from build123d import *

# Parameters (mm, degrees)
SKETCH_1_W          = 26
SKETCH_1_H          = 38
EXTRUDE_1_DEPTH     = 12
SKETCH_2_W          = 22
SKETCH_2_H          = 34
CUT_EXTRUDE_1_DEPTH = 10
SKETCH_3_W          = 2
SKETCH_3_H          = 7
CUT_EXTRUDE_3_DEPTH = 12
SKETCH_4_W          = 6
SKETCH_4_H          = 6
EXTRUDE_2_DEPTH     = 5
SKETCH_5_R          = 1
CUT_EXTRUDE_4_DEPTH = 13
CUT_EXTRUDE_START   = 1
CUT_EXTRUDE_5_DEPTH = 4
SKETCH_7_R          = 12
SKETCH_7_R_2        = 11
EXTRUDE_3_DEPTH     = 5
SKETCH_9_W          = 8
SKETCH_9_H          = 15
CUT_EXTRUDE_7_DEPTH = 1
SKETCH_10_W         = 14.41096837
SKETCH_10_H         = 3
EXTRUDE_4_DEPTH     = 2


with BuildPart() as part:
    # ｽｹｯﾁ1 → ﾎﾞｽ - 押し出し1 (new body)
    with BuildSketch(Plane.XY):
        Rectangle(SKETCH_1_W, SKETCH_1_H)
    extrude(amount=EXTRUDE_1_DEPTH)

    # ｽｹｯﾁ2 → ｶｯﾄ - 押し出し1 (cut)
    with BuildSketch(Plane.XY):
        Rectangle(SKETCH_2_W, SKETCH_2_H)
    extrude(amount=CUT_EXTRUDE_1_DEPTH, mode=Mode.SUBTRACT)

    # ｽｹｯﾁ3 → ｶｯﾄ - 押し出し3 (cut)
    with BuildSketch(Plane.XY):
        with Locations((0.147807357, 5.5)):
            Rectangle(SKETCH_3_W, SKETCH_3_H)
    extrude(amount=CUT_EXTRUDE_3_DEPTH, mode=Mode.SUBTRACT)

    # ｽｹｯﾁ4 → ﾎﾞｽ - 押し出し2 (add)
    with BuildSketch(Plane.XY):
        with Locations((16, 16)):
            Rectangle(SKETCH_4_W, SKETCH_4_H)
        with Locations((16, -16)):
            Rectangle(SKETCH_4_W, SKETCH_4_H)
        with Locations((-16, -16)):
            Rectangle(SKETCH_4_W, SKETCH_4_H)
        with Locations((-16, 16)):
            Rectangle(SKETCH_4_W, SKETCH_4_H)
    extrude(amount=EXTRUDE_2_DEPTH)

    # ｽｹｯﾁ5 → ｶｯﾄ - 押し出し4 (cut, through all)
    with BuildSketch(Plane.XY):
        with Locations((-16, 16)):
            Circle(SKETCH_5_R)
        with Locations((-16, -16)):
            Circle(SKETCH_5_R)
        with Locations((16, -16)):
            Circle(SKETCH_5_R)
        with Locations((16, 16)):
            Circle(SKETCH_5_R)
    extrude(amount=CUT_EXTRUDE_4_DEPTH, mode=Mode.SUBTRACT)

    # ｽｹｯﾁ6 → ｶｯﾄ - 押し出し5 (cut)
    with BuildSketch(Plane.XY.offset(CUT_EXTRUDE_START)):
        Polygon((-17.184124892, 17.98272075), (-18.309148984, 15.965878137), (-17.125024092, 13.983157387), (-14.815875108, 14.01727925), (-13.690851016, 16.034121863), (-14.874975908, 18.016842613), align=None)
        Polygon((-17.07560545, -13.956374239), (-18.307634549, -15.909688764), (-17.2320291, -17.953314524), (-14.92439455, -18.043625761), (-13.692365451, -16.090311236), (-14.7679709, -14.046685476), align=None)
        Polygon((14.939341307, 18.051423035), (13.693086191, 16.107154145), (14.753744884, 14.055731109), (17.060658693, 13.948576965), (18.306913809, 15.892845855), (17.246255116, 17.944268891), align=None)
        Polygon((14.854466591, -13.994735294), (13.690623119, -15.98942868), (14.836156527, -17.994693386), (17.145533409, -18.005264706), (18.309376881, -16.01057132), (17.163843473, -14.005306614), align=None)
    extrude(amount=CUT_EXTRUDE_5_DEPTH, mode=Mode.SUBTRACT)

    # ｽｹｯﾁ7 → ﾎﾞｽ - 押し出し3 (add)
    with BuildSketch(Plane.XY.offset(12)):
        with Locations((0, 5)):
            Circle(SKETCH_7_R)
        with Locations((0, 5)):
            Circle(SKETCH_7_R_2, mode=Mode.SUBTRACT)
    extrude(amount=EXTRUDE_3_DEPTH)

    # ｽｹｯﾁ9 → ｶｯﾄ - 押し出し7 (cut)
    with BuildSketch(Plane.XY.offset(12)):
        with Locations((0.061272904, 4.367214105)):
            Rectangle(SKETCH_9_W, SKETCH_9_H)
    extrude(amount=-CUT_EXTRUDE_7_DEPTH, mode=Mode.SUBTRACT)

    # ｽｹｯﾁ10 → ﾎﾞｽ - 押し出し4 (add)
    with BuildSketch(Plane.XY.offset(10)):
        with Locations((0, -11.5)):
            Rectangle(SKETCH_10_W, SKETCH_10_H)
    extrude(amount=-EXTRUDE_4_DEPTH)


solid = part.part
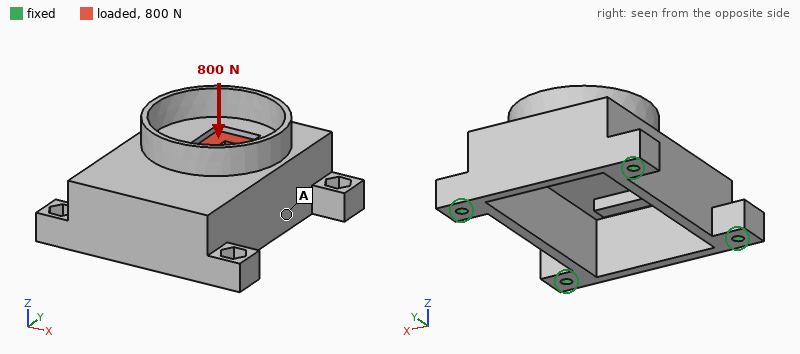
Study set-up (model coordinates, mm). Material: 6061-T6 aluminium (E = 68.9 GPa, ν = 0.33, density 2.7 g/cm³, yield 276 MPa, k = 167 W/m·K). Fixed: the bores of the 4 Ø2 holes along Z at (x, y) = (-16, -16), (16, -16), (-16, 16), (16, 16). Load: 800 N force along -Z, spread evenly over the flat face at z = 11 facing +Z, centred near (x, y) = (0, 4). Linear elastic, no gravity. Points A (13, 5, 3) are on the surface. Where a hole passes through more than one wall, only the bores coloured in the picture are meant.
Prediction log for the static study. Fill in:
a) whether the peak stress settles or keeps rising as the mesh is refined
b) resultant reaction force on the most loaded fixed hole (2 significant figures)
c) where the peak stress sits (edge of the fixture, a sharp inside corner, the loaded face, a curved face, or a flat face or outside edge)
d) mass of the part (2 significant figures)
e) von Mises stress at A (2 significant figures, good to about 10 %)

keeps rising
320 N
a sharp inside corner
14 g
22 MPa
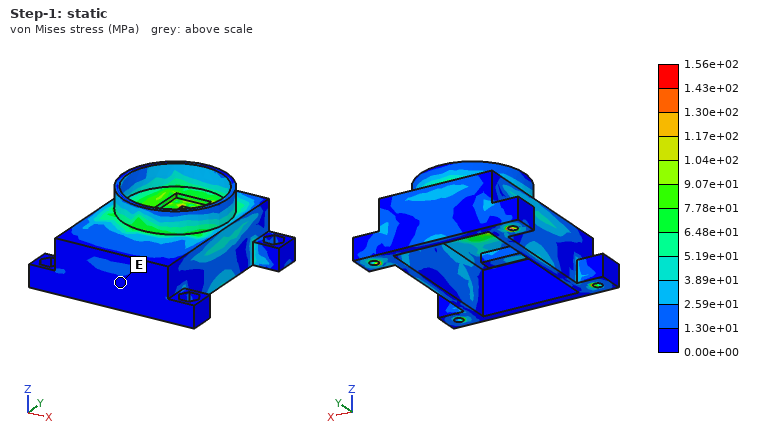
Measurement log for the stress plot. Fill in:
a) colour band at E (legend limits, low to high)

0.00e+00 to 1.30e+01 MPa
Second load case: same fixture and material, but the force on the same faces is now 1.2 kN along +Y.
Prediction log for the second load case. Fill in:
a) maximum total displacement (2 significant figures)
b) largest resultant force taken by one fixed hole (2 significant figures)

25 µm
360 N
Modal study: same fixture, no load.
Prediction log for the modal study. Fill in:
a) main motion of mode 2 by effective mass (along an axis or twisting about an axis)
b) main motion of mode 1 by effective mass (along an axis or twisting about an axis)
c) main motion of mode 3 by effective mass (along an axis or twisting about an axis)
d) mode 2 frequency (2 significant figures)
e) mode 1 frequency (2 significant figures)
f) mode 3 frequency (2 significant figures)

along Z
along Y
along X
13 kHz
12 kHz
15 kHz
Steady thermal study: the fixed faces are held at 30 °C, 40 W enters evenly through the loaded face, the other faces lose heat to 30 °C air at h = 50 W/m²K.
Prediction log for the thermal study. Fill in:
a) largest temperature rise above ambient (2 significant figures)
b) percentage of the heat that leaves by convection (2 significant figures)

59 K
19 %
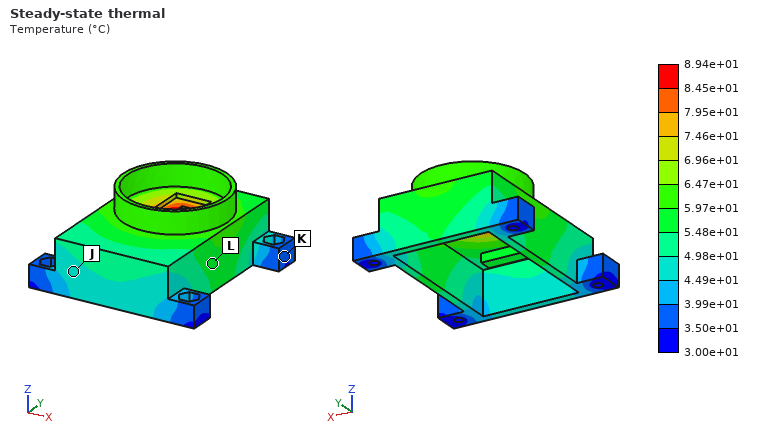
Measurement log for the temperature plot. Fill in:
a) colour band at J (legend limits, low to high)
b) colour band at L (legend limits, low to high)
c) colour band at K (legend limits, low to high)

4.49e+01 to 4.98e+01 °C
5.48e+01 to 5.97e+01 °C
3.50e+01 to 3.99e+01 °C
